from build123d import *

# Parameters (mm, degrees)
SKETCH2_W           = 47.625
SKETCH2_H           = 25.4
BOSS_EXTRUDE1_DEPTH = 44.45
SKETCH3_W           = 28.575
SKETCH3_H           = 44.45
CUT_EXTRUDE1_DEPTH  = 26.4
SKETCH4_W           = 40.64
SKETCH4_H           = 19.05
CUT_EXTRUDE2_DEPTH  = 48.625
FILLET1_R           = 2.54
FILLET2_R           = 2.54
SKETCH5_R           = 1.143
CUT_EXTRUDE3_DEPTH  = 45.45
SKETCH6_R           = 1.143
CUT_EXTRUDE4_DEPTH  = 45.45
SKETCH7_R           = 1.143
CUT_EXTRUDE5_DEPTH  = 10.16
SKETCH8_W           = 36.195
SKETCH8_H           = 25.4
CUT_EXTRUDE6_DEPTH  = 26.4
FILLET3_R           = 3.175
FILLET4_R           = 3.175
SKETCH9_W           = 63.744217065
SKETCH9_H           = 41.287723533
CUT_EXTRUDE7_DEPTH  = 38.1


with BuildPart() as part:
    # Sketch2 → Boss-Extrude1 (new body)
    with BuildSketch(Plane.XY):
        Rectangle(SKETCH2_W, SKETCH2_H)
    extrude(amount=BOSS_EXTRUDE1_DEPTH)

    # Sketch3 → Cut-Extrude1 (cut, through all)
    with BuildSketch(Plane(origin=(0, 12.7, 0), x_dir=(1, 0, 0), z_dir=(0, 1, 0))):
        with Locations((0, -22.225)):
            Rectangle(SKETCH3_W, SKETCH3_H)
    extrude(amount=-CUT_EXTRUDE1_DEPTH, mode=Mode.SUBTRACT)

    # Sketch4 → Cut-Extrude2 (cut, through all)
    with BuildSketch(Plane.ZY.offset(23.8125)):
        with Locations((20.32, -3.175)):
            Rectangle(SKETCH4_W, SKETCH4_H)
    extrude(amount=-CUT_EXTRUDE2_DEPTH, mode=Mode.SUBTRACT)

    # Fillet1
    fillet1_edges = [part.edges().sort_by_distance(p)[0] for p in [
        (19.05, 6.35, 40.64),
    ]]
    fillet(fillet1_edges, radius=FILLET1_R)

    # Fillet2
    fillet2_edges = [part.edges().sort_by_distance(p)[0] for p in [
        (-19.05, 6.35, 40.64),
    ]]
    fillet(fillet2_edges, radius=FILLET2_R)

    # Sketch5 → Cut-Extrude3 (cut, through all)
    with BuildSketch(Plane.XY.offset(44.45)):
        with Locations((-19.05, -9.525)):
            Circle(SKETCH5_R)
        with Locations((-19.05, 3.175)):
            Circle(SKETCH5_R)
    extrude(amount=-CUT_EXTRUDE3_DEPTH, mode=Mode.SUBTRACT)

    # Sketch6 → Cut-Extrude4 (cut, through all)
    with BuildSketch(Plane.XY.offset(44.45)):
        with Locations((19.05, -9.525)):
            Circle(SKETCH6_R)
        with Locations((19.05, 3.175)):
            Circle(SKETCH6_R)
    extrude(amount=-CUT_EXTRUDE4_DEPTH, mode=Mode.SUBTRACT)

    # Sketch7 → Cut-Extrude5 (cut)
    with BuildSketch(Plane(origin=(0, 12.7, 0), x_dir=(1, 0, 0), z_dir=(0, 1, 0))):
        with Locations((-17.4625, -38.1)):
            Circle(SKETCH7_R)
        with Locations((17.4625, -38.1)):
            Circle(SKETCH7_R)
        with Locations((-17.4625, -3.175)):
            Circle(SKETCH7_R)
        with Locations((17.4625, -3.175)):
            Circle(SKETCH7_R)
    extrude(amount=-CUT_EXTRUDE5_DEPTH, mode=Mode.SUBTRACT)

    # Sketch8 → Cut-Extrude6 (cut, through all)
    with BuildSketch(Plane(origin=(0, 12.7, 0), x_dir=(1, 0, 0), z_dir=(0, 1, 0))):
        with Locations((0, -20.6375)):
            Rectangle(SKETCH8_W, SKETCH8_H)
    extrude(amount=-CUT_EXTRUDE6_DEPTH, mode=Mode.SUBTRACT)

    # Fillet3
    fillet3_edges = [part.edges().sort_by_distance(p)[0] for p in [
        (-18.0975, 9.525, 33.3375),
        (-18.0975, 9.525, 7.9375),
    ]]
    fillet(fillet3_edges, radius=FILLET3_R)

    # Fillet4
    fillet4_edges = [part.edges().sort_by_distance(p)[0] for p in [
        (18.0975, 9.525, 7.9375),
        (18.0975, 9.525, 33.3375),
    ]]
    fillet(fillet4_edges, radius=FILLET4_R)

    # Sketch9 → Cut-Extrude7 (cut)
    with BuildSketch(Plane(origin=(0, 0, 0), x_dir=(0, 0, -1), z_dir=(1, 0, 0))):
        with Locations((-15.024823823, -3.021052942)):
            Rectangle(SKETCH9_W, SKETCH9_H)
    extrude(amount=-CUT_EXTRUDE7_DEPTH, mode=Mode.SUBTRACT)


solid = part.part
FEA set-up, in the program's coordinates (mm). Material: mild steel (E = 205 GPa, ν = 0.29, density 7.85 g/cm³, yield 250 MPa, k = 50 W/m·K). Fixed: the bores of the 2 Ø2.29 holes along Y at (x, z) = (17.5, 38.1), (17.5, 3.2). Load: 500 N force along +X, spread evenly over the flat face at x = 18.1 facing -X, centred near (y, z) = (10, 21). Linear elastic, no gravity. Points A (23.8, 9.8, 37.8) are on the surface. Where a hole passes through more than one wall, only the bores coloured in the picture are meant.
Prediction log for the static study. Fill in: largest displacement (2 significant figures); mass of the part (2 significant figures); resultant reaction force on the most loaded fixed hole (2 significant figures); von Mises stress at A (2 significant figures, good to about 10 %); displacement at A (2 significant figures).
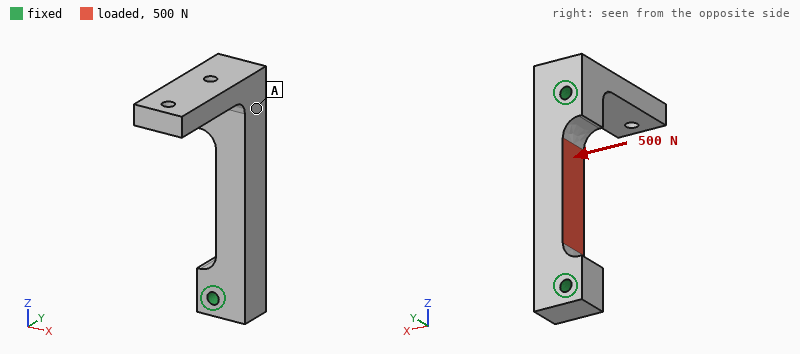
4.3 µm
21 g
370 N
8.2 MPa
0.88 µm
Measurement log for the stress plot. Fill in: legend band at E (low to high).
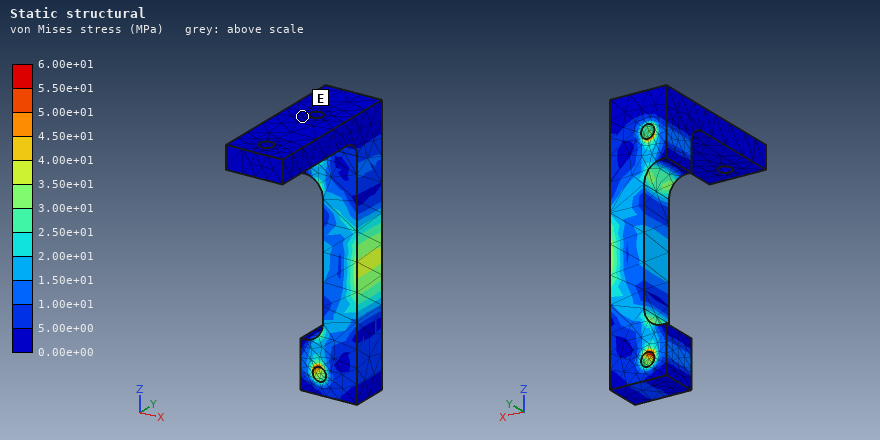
0.00e+00 to 5.00e+00 MPa
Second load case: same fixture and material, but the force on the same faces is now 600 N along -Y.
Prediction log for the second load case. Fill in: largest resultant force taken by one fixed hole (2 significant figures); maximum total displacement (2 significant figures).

300 N
6.9 µm
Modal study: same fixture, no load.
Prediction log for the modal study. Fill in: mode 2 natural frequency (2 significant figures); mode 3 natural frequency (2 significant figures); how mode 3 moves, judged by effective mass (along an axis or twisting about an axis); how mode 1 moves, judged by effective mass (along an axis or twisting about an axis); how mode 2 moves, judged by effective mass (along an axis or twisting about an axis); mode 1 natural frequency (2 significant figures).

11 kHz
23 kHz
along Y
along Z
along X
7200 Hz
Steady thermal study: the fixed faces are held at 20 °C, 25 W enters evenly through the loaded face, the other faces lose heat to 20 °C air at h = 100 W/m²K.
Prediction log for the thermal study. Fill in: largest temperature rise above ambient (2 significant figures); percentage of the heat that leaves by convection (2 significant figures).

80 K
13 %
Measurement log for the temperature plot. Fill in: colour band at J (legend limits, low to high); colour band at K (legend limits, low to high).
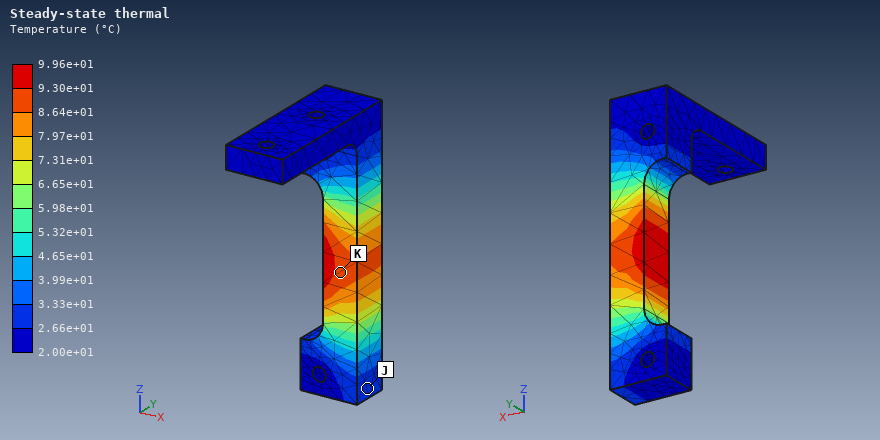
2.66e+01 to 3.33e+01 °C
8.64e+01 to 9.30e+01 °C
